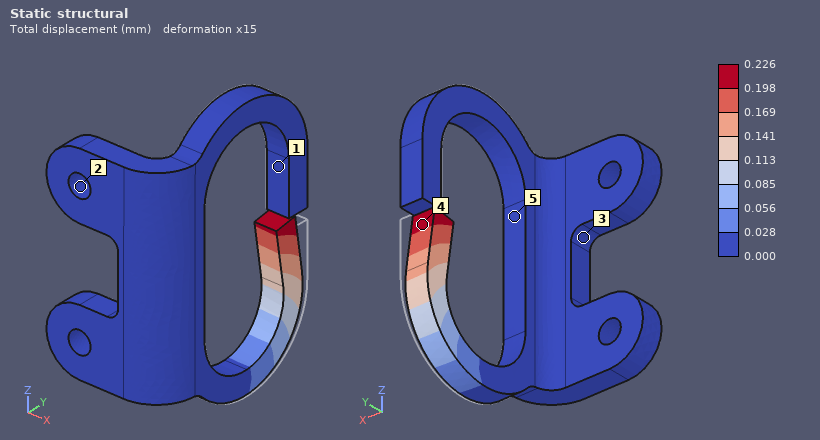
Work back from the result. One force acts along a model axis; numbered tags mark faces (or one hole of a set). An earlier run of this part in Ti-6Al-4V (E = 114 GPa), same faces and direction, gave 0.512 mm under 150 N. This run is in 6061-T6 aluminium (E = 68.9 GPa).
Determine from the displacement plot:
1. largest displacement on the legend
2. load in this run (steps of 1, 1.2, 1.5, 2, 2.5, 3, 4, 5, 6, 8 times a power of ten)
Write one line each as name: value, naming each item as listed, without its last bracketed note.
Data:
largest displacement on the legend: 0.226 mm
load in this run: 40 N
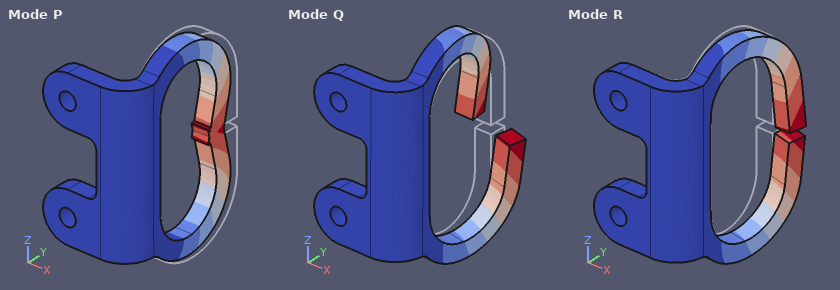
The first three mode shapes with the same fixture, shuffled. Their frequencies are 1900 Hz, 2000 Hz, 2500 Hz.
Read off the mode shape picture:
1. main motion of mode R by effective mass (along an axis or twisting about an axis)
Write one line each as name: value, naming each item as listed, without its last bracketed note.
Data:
main motion of mode R by effective mass: along X
